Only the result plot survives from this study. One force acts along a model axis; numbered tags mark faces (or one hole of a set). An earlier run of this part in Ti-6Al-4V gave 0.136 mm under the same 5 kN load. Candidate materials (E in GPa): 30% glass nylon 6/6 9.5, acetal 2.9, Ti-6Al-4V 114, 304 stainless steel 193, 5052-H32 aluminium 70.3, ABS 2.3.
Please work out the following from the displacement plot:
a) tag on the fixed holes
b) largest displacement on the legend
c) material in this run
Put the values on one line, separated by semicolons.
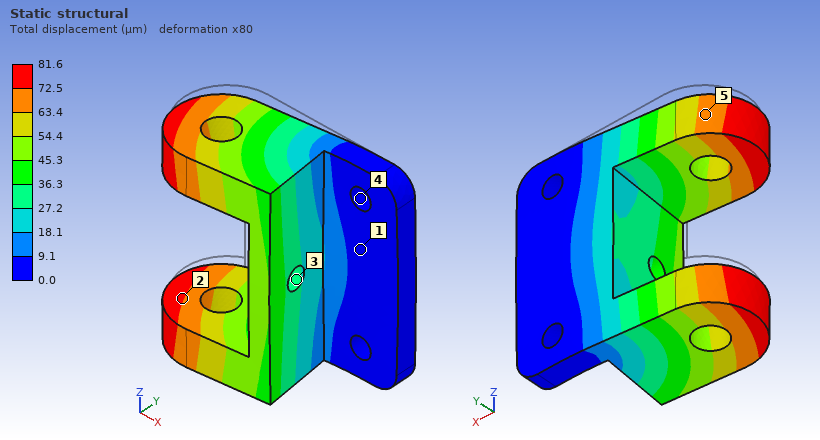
4; 81.6 µm; 304 stainless steel
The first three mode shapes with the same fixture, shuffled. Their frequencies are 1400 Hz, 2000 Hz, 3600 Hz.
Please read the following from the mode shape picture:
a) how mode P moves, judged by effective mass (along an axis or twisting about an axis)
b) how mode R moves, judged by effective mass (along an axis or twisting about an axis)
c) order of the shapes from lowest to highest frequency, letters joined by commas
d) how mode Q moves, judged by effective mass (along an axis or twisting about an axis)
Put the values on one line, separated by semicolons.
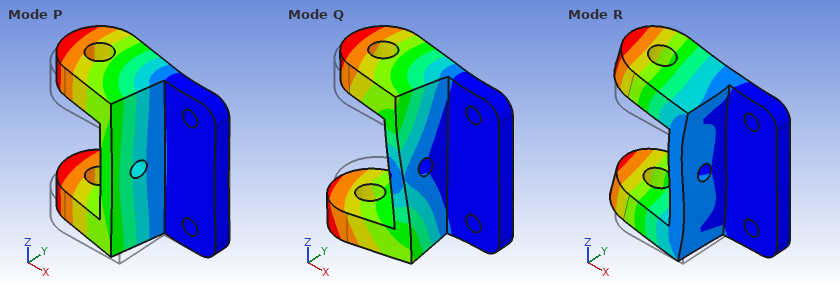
along Y; along Z; P, Q, R; twisting about X
